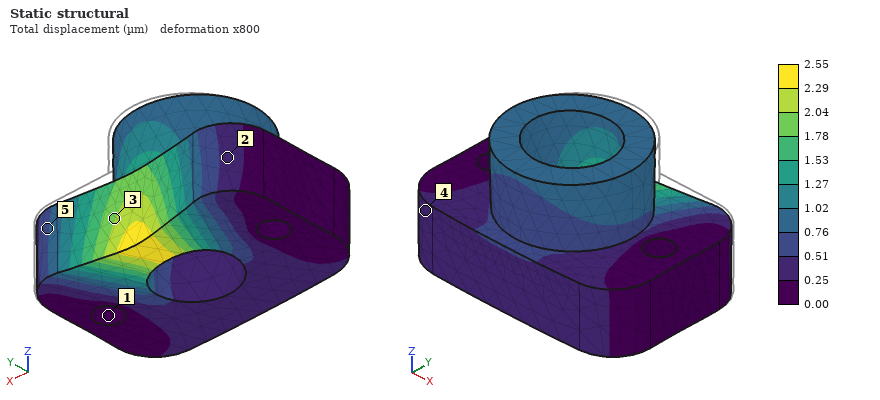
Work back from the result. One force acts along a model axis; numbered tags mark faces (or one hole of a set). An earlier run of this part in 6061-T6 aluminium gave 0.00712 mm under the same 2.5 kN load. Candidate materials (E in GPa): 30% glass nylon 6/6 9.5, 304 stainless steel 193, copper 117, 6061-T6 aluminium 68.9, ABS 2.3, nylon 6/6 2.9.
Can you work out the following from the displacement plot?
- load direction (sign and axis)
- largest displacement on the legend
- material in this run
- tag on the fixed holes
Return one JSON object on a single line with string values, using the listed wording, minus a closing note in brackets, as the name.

{"load direction": "-Y", "largest displacement on the legend": "2.55 µm", "material in this run": "304 stainless steel", "tag on the fixed holes": "1"}
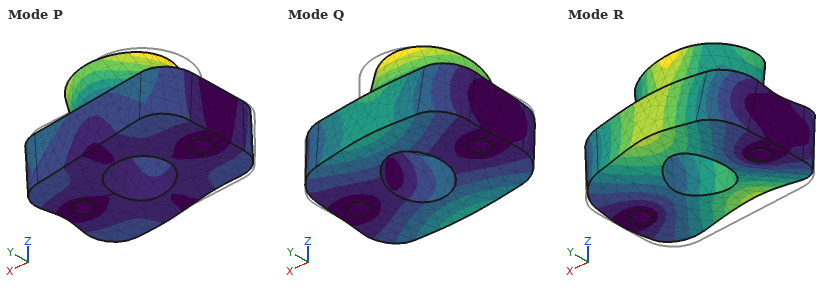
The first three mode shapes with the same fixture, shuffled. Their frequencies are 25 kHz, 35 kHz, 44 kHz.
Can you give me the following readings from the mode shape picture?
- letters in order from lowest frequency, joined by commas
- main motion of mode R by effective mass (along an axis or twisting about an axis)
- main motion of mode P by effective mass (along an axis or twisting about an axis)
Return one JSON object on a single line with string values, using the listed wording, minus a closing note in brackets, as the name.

{"letters in order from lowest frequency, joined by commas": "Q, R, P", "main motion of mode R by effective mass": "along Z", "main motion of mode P by effective mass": "along X"}
